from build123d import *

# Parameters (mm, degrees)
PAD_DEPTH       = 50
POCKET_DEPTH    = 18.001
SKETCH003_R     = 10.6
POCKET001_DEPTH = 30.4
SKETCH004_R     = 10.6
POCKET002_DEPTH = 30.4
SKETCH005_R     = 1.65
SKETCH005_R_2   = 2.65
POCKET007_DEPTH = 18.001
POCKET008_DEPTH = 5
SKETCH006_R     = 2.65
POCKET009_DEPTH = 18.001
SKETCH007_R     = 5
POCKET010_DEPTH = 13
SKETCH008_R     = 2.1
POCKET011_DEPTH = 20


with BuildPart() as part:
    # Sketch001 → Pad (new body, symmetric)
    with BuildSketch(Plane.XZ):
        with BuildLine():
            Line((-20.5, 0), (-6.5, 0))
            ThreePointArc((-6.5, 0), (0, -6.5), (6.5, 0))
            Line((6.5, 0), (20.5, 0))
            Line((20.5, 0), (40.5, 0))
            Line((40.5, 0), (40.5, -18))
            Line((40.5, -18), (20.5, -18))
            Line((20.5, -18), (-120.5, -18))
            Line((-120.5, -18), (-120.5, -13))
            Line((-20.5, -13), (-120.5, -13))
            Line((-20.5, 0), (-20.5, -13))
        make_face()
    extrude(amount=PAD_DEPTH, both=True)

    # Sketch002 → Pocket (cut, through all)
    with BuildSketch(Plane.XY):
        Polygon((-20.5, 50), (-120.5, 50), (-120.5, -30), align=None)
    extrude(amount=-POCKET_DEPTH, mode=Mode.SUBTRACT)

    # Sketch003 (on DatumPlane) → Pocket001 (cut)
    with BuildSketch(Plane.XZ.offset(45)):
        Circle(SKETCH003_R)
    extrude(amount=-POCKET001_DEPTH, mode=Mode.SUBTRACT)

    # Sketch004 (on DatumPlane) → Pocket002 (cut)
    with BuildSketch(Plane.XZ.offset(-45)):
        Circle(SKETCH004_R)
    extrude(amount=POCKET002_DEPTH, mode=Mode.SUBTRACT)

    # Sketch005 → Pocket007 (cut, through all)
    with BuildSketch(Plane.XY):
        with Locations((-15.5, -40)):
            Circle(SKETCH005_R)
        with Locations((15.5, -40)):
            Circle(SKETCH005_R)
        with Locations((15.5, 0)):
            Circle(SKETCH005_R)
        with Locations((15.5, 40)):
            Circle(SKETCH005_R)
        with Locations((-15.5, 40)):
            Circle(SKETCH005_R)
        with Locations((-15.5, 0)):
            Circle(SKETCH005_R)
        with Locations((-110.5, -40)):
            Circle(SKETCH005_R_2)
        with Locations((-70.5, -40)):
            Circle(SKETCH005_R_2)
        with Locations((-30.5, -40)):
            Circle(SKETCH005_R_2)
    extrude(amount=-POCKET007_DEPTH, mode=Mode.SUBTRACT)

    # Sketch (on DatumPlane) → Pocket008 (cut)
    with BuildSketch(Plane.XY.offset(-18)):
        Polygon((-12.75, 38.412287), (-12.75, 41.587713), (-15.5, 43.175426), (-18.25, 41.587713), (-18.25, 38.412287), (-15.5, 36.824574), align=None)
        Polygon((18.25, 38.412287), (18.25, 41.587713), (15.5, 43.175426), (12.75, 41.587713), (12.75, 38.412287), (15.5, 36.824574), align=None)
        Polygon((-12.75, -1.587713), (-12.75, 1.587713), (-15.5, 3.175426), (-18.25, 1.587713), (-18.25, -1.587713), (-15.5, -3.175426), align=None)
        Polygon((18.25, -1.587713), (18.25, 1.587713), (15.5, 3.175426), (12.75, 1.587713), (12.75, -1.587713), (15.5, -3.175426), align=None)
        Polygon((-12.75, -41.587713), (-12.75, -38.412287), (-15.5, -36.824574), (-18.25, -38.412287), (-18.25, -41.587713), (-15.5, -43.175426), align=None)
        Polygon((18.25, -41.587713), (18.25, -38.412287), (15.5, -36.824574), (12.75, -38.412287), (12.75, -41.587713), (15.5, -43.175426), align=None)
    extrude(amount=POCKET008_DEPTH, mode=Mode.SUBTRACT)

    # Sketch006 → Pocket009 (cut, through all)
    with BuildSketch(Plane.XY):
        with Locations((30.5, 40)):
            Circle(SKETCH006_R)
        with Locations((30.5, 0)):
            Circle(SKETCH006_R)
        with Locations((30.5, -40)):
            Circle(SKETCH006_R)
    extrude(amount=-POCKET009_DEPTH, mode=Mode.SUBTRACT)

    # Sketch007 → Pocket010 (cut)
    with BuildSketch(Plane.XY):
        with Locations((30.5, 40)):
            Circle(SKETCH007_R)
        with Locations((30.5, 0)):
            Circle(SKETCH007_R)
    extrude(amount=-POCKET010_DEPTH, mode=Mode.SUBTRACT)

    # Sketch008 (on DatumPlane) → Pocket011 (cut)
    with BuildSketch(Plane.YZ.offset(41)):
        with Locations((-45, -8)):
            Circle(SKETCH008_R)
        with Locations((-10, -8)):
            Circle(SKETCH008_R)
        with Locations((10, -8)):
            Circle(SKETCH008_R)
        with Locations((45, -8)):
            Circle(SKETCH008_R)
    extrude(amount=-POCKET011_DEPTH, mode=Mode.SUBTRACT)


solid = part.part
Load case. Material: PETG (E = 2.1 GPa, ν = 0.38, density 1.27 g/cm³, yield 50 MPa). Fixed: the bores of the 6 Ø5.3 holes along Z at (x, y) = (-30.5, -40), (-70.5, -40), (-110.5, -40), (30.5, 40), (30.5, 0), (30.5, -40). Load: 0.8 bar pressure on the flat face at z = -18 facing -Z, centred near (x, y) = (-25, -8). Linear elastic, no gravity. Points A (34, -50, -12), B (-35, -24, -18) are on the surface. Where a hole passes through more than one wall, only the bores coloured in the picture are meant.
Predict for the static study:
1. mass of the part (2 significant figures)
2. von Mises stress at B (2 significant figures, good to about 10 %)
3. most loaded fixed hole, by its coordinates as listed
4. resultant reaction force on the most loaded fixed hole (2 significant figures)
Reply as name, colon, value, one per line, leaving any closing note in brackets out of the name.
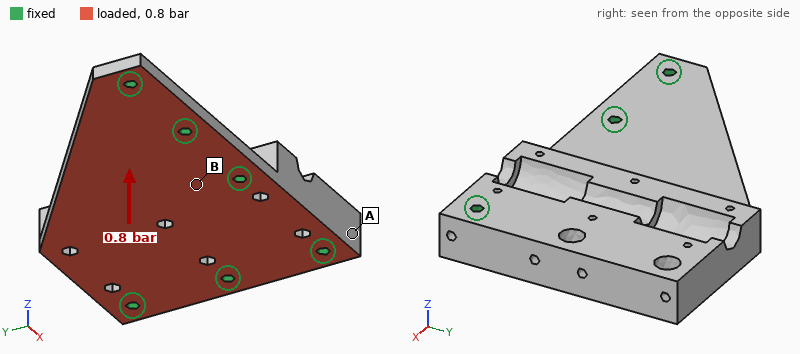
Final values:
mass of the part: 150 g
von Mises stress at B: 3.4 MPa
most loaded fixed hole, by its coordinates as listed: (-30.5, -40)
resultant reaction force on the most loaded fixed hole: 360 N
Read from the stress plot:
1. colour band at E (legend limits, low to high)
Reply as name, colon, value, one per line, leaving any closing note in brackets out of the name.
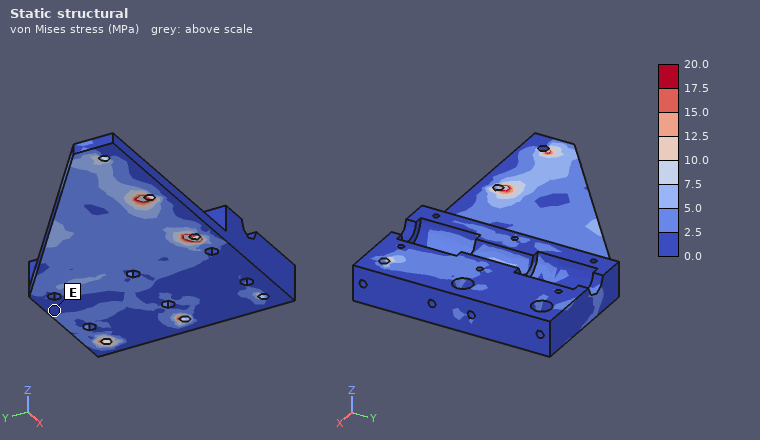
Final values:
colour band at E: 0.0 to 2.5 MPa
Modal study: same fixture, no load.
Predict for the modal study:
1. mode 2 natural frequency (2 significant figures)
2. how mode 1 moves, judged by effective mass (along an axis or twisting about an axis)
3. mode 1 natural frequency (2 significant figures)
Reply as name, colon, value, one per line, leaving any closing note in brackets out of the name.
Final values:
mode 2 natural frequency: 950 Hz
how mode 1 moves, judged by effective mass: along Z
mode 1 natural frequency: 600 Hz
